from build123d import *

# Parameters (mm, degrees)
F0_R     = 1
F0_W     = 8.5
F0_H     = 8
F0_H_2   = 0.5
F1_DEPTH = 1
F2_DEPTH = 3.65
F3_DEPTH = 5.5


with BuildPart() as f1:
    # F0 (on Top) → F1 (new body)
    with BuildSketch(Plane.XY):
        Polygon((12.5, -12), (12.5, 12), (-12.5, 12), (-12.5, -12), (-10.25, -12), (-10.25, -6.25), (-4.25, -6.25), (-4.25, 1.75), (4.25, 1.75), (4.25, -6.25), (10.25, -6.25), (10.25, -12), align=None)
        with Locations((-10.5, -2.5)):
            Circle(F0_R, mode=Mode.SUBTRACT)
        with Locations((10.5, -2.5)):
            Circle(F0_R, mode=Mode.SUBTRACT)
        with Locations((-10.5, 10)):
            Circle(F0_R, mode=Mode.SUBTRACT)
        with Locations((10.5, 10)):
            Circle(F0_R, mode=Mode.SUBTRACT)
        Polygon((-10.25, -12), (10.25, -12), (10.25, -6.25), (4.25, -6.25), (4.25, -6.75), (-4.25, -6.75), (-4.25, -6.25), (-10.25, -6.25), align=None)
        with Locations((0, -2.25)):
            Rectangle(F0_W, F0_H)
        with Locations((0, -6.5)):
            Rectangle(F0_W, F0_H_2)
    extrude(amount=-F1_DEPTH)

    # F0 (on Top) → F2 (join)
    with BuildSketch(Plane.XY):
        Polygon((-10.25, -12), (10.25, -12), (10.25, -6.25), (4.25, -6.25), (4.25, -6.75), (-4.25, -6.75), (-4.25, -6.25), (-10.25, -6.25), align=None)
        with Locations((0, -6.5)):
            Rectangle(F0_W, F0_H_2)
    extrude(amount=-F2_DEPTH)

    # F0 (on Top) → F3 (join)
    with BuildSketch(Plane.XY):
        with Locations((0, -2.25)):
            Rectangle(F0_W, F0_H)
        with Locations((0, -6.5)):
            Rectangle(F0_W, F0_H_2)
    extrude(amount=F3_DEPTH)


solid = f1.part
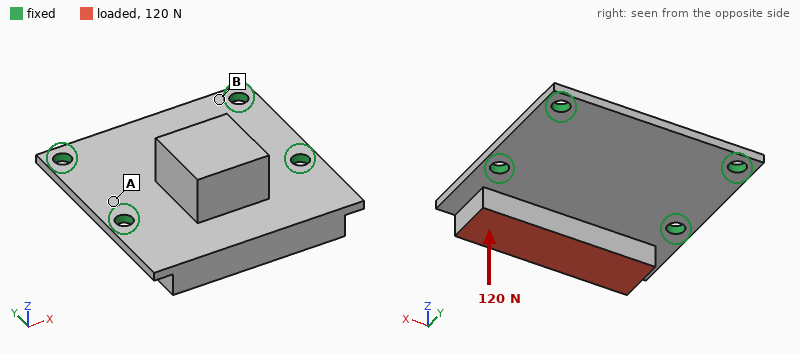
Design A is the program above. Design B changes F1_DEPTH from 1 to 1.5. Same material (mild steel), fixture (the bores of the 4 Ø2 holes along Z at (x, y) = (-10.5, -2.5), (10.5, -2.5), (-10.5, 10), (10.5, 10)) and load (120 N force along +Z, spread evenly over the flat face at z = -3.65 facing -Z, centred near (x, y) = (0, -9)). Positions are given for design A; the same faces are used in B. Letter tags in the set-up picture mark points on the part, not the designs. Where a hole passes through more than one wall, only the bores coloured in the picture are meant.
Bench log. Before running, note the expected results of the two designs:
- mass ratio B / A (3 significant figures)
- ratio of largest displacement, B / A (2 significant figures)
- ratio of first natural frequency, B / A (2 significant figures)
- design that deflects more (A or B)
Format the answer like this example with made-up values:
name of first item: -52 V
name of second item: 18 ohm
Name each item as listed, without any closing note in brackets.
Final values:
mass ratio B / A: 1.18
ratio of largest displacement, B / A: 0.41
ratio of first natural frequency, B / A: 1.5
design that deflects more: A
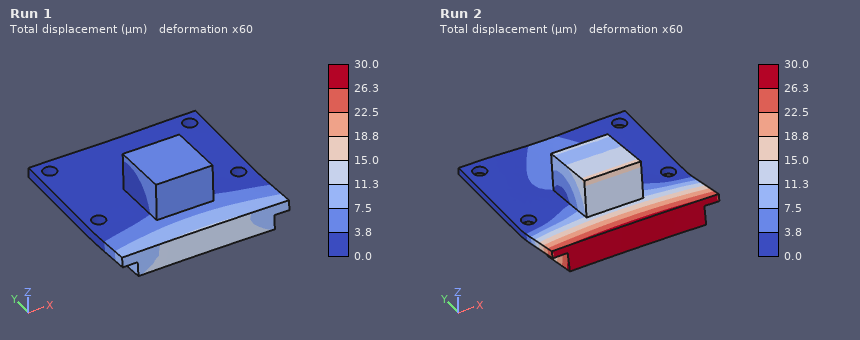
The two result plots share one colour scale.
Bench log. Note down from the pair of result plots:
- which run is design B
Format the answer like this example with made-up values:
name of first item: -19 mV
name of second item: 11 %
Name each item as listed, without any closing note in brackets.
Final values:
which run is design B: Run 1
